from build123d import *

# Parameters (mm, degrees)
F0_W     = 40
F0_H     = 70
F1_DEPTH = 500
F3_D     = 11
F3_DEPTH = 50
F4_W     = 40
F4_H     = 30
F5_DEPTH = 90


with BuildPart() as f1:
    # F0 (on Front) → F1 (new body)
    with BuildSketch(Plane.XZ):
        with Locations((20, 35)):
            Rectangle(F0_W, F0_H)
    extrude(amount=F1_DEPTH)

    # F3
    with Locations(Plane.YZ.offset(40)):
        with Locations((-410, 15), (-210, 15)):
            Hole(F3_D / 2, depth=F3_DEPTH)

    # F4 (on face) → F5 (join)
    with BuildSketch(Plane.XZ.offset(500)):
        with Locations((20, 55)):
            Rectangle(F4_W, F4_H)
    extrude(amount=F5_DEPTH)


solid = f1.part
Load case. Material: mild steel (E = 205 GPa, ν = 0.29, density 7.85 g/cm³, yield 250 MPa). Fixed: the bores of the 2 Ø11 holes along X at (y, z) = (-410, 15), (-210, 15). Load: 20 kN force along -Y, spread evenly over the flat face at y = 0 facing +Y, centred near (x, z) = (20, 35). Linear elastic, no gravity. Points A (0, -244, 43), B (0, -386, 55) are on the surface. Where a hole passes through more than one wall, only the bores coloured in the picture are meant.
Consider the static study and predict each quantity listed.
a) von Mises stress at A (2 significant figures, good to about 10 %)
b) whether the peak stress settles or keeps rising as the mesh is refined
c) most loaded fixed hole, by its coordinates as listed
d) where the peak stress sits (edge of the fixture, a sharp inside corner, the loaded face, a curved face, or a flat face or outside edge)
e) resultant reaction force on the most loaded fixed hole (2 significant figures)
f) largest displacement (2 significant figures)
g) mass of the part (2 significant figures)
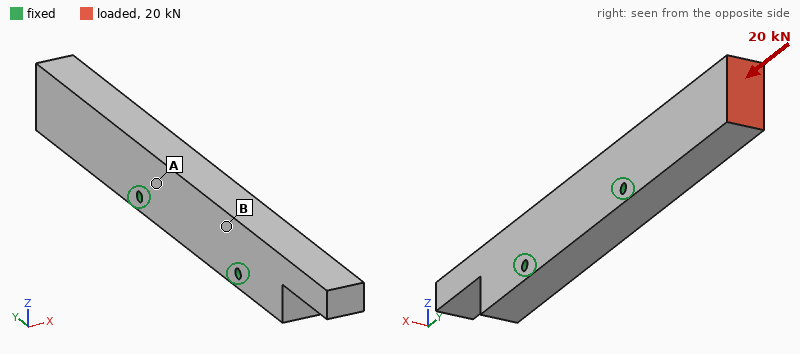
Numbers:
3.5 MPa
keeps rising
(-210, 15)
edge of the fixture
16 kN
19 µm
12 kg
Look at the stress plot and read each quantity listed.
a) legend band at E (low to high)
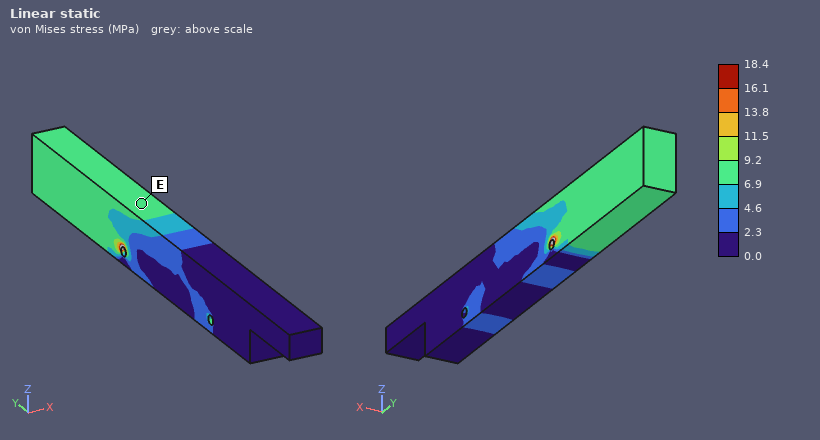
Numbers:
6.9 to 9.2 MPa
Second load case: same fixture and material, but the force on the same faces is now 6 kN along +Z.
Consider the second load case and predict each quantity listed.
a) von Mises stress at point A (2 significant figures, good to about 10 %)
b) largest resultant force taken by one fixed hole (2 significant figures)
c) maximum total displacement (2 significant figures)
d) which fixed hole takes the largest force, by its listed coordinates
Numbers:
9.2 MPa
16 kN
0.13 mm
(-210, 15)
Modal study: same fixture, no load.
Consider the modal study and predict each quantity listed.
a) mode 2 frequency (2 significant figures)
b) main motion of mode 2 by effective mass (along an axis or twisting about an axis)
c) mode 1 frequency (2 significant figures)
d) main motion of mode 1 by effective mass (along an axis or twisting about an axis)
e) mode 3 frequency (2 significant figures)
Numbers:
940 Hz
along Z
660 Hz
along X
1200 Hz
